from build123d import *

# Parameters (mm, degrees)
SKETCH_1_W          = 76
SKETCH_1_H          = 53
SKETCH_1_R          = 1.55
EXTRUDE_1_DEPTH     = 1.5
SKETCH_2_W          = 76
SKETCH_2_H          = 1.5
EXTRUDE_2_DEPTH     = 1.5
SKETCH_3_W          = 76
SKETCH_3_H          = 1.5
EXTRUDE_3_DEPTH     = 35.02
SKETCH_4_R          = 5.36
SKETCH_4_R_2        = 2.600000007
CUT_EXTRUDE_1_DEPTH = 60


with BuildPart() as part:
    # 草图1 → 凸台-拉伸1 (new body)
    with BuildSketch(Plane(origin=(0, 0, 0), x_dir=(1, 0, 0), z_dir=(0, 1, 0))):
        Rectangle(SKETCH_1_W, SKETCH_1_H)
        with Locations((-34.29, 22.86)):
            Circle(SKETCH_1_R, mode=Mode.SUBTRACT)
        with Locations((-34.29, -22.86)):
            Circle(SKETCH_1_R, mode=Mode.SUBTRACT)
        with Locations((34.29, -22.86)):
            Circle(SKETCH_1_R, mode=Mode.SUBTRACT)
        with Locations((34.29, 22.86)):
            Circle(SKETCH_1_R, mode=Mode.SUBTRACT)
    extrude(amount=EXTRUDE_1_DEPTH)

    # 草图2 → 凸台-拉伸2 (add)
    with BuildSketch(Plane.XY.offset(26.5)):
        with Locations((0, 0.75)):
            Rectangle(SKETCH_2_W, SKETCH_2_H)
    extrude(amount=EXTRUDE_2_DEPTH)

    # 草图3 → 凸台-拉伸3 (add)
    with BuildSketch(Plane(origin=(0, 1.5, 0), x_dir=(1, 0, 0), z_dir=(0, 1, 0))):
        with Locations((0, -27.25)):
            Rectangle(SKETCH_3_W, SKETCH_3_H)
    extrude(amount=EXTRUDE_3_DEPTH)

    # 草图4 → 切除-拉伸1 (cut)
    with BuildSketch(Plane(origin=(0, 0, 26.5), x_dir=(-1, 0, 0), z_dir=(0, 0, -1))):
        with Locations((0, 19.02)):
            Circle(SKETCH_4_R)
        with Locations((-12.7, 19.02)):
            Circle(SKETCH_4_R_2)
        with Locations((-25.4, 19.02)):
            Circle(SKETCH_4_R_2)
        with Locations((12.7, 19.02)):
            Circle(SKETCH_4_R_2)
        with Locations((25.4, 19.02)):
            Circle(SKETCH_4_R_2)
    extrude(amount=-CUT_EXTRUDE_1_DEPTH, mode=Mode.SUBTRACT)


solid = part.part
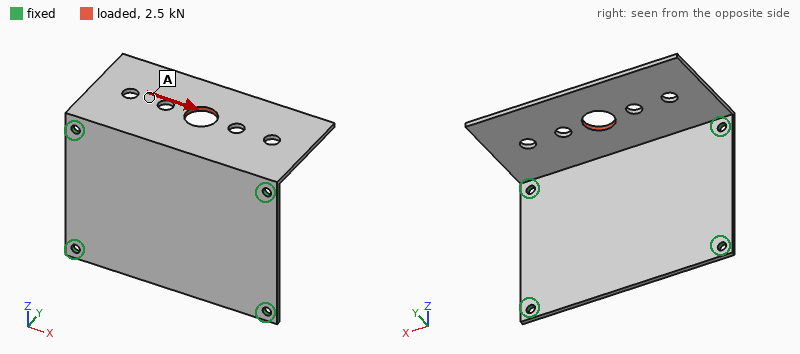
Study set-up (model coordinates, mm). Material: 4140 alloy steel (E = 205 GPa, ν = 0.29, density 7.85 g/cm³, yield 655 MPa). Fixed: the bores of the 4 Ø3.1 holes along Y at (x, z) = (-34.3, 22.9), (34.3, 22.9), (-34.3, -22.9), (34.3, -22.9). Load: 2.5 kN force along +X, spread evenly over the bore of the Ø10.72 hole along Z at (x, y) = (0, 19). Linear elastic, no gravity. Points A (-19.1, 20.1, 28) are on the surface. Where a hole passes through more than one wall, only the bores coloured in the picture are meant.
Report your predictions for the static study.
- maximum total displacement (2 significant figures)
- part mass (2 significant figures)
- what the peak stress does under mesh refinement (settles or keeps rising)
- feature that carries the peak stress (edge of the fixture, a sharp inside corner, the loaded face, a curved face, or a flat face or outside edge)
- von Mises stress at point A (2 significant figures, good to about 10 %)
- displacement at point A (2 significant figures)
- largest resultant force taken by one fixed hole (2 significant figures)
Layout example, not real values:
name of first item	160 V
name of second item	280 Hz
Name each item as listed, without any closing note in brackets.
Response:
maximum total displacement	0.10 mm
part mass	78 g
what the peak stress does under mesh refinement	keeps rising
feature that carries the peak stress	edge of the fixture
von Mises stress at point A	39 MPa
displacement at point A	0.038 mm
largest resultant force taken by one fixed hole	1.3 kN
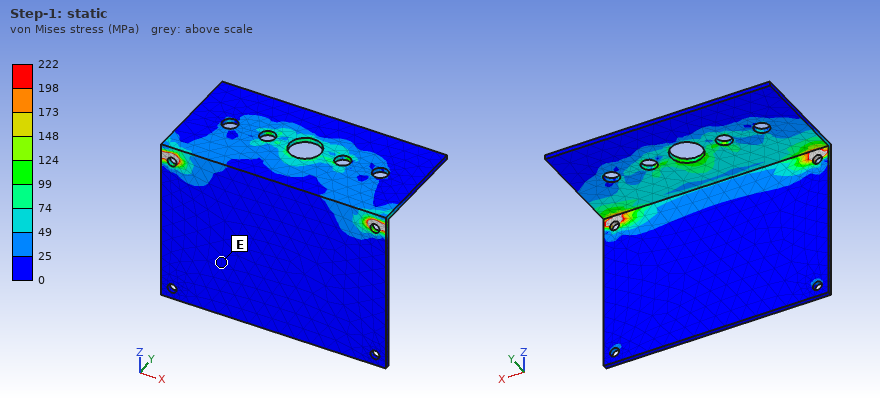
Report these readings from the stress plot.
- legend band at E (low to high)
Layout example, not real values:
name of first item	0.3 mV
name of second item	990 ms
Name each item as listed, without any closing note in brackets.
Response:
legend band at E	0 to 25 MPa
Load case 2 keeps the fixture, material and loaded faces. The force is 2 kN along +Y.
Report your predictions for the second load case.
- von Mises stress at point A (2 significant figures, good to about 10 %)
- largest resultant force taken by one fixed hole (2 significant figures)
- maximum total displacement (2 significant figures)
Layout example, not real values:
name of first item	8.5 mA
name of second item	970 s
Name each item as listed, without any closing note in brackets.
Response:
von Mises stress at point A	61 MPa
largest resultant force taken by one fixed hole	1.2 kN
maximum total displacement	0.23 mm
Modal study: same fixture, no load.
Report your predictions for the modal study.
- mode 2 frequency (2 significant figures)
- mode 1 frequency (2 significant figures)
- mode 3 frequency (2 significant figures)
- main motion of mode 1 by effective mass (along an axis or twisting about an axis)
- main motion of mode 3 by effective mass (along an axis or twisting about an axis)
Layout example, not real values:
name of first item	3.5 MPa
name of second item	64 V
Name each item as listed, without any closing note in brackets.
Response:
mode 2 frequency	1300 Hz
mode 1 frequency	730 Hz
mode 3 frequency	1700 Hz
main motion of mode 1 by effective mass	along Z
main motion of mode 3 by effective mass	along Y
